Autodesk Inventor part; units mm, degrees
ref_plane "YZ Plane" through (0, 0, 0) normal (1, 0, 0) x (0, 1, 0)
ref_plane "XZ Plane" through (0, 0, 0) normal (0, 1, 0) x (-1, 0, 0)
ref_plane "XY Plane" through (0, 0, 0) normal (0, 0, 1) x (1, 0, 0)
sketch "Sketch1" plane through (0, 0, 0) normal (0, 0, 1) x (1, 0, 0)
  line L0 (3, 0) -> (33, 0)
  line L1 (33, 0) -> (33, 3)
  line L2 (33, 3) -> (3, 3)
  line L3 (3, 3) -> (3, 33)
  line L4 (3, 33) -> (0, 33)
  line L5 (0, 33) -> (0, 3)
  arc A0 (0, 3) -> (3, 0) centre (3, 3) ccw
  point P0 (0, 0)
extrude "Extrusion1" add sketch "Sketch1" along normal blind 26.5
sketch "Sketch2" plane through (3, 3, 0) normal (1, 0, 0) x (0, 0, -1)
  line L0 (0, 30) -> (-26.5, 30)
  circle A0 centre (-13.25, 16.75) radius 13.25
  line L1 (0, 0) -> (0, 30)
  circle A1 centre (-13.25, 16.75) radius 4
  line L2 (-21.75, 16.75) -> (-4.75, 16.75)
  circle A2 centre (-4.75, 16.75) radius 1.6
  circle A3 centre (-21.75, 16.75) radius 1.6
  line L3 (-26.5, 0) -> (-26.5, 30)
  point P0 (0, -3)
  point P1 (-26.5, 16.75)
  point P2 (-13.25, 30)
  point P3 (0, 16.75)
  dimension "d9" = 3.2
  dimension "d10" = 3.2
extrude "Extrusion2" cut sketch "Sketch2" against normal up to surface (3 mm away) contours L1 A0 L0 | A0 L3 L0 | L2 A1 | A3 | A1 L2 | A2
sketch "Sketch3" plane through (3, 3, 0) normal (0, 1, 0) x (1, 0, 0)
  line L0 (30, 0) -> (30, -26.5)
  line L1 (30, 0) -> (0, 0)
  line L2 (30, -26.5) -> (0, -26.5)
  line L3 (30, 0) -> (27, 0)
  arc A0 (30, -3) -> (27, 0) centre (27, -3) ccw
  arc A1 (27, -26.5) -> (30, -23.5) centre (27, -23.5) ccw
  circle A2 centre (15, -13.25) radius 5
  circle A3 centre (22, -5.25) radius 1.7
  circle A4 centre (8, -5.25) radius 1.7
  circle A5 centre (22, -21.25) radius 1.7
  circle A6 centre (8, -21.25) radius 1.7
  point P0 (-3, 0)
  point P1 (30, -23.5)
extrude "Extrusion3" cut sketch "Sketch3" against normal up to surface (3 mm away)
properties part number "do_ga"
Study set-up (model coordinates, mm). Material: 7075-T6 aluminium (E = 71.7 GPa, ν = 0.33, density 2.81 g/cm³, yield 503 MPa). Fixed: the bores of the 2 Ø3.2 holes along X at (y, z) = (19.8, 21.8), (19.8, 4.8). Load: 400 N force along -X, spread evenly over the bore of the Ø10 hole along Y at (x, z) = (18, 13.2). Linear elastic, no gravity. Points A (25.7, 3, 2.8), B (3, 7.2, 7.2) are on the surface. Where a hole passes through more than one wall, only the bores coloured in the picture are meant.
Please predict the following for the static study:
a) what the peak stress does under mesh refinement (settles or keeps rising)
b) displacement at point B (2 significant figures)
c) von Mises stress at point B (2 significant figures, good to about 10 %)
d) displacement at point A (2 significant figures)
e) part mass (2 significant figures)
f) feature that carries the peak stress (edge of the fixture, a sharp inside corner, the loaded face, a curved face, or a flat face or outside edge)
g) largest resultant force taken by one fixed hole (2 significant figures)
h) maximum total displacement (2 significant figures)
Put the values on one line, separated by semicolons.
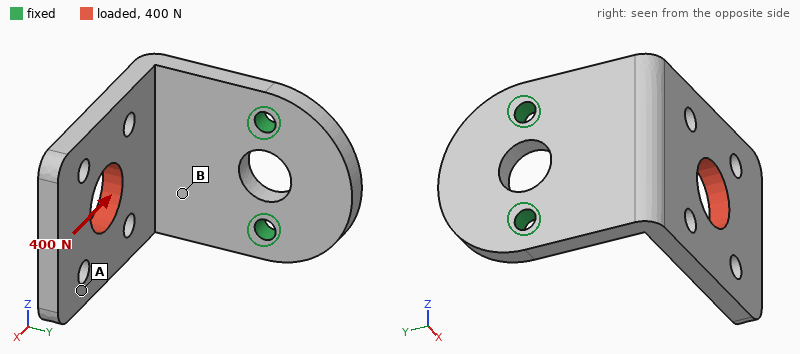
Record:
keeps rising; 0.12 mm; 53 MPa; 0.44 mm; 12 g; edge of the fixture; 200 N; 0.57 mm
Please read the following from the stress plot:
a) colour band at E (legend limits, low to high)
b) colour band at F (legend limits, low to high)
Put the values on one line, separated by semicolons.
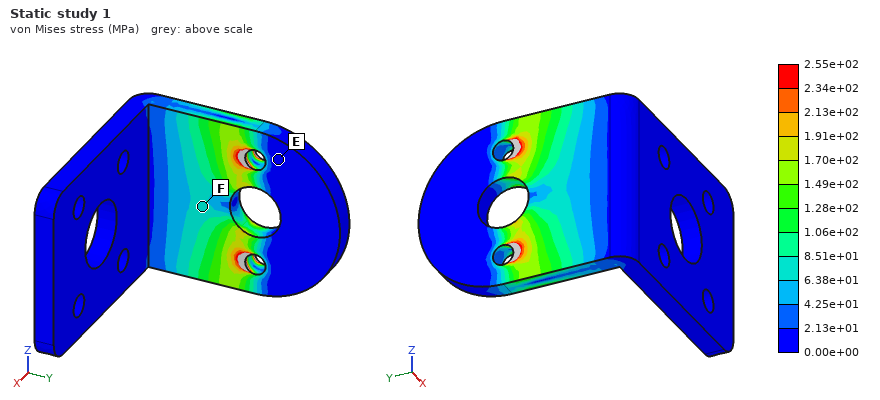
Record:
0.00e+00 to 2.13e+01 MPa; 6.38e+01 to 8.51e+01 MPa
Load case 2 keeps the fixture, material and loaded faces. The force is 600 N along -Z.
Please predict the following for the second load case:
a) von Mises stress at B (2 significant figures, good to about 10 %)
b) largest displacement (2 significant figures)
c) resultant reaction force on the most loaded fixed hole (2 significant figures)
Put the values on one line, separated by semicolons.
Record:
160 MPa; 0.54 mm; 790 N
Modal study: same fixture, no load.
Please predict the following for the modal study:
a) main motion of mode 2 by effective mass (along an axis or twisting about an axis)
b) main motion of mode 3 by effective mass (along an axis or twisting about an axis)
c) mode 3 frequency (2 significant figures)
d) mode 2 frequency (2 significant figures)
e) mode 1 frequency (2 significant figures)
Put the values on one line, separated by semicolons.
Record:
along Z; along X; 4000 Hz; 2500 Hz; 1300 Hz
